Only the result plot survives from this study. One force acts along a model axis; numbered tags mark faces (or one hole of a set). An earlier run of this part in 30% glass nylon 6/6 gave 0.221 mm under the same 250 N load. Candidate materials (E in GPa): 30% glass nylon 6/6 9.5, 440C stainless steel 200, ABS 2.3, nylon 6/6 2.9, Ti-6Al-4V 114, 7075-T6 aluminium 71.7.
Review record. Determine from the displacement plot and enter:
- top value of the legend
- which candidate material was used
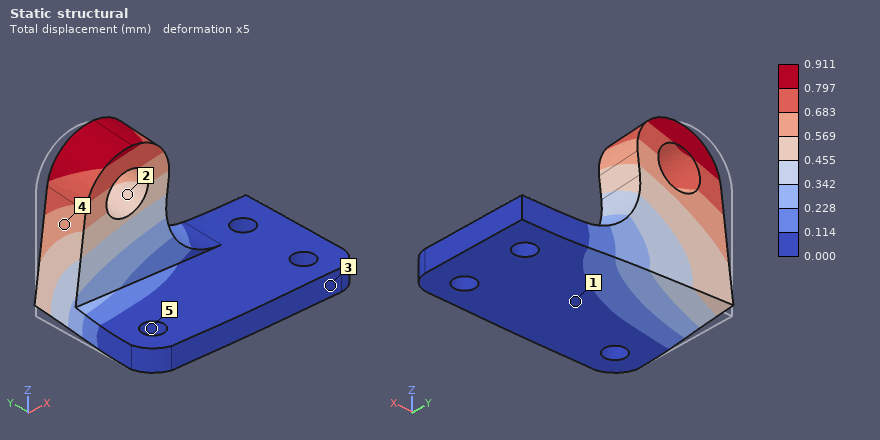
0.911 mm
ABS
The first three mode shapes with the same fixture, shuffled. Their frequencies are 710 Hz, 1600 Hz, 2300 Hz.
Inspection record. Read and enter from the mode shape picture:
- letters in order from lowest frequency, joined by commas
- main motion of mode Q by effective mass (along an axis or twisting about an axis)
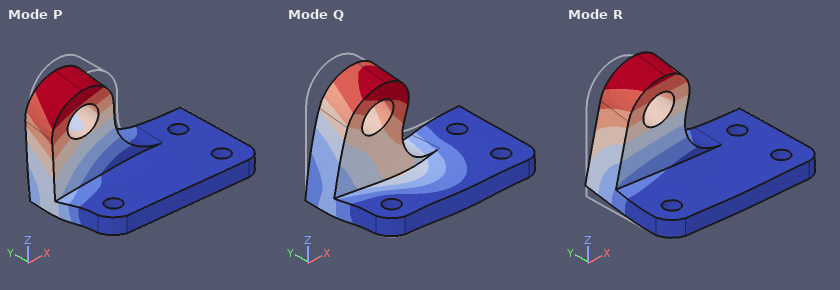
R, P, Q
along Z
